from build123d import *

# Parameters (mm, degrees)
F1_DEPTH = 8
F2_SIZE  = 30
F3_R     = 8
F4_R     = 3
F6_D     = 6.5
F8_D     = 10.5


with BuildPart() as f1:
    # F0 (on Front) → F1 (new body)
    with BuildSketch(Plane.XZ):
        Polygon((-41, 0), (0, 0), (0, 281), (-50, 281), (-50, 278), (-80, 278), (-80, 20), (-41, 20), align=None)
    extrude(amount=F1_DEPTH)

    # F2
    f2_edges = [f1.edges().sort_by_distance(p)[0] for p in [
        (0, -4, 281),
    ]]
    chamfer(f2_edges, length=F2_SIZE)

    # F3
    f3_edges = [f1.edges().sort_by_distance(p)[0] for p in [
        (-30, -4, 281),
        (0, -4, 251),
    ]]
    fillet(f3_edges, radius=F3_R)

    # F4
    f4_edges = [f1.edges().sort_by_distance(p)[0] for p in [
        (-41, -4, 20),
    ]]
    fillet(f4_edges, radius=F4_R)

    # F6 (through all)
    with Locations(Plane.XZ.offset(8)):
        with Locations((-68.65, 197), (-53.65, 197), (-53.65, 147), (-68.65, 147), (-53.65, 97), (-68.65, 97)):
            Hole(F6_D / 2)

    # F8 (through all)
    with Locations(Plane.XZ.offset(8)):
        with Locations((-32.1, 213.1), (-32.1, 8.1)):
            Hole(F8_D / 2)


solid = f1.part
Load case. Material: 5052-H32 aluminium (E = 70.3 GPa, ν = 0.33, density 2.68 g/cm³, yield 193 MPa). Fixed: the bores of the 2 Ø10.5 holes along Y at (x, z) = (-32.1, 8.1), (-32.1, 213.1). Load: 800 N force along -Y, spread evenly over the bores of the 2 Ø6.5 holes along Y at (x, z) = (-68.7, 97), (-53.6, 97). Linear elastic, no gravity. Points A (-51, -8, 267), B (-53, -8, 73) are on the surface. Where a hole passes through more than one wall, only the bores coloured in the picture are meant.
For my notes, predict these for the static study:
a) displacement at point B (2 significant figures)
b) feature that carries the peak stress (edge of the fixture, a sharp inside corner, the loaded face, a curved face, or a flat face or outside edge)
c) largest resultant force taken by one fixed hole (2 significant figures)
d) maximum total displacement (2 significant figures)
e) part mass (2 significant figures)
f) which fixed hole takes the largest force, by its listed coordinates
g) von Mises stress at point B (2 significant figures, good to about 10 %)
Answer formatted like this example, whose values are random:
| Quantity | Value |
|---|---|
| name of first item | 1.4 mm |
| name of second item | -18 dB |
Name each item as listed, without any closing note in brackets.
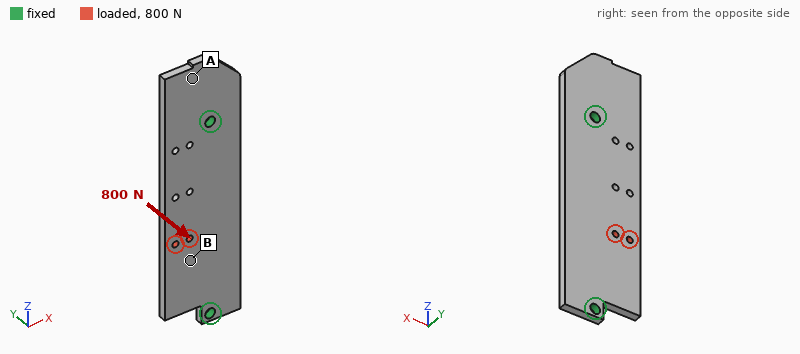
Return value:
| Quantity | Value |
|---|---|
| displacement at point B | 0.21 mm |
| feature that carries the peak stress | a curved face |
| largest resultant force taken by one fixed hole | 450 N |
| maximum total displacement | 0.35 mm |
| part mass | 450 g |
| which fixed hole takes the largest force, by its listed coordinates | (-32.1, 8.1) |
| von Mises stress at point B | 16 MPa |
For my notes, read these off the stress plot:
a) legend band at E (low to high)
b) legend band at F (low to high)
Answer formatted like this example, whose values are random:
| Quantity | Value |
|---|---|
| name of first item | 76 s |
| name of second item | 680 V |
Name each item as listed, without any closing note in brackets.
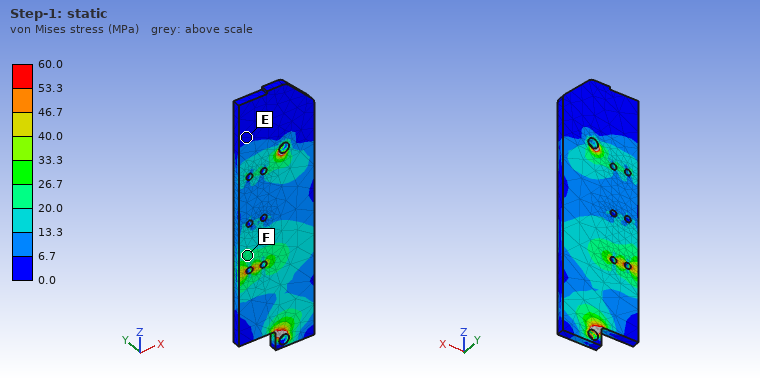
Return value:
| Quantity | Value |
|---|---|
| legend band at E | 0.0 to 6.7 MPa |
| legend band at F | 20.0 to 26.7 MPa |
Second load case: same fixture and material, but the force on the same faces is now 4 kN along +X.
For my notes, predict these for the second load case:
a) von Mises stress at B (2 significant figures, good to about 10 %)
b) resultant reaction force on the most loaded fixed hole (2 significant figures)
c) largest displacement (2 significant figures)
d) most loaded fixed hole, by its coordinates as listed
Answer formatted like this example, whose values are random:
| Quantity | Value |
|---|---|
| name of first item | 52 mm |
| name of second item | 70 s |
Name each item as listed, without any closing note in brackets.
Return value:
| Quantity | Value |
|---|---|
| von Mises stress at B | 11 MPa |
| resultant reaction force on the most loaded fixed hole | 2.4 kN |
| largest displacement | 42 µm |
| most loaded fixed hole, by its coordinates as listed | (-32.1, 8.1) |
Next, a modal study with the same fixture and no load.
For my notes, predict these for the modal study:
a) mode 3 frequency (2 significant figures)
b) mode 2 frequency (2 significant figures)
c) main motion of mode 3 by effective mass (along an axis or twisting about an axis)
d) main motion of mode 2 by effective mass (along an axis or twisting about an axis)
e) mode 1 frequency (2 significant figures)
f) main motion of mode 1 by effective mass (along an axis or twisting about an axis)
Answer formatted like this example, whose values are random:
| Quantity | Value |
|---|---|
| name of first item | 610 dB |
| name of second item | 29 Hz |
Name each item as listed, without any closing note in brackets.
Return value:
| Quantity | Value |
|---|---|
| mode 3 frequency | 1500 Hz |
| mode 2 frequency | 1300 Hz |
| main motion of mode 3 by effective mass | along Y |
| main motion of mode 2 by effective mass | twisting about Z |
| mode 1 frequency | 850 Hz |
| main motion of mode 1 by effective mass | along Y |
